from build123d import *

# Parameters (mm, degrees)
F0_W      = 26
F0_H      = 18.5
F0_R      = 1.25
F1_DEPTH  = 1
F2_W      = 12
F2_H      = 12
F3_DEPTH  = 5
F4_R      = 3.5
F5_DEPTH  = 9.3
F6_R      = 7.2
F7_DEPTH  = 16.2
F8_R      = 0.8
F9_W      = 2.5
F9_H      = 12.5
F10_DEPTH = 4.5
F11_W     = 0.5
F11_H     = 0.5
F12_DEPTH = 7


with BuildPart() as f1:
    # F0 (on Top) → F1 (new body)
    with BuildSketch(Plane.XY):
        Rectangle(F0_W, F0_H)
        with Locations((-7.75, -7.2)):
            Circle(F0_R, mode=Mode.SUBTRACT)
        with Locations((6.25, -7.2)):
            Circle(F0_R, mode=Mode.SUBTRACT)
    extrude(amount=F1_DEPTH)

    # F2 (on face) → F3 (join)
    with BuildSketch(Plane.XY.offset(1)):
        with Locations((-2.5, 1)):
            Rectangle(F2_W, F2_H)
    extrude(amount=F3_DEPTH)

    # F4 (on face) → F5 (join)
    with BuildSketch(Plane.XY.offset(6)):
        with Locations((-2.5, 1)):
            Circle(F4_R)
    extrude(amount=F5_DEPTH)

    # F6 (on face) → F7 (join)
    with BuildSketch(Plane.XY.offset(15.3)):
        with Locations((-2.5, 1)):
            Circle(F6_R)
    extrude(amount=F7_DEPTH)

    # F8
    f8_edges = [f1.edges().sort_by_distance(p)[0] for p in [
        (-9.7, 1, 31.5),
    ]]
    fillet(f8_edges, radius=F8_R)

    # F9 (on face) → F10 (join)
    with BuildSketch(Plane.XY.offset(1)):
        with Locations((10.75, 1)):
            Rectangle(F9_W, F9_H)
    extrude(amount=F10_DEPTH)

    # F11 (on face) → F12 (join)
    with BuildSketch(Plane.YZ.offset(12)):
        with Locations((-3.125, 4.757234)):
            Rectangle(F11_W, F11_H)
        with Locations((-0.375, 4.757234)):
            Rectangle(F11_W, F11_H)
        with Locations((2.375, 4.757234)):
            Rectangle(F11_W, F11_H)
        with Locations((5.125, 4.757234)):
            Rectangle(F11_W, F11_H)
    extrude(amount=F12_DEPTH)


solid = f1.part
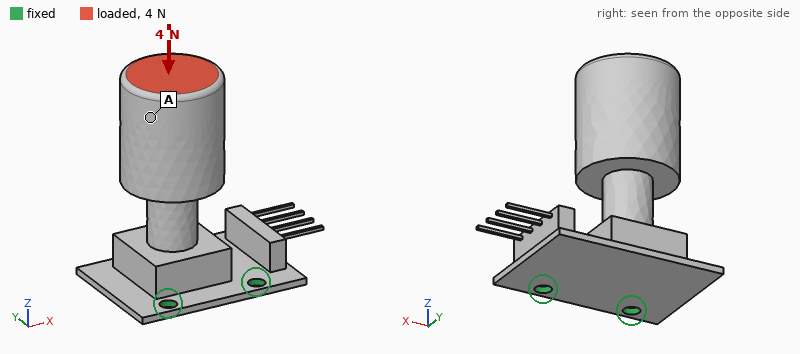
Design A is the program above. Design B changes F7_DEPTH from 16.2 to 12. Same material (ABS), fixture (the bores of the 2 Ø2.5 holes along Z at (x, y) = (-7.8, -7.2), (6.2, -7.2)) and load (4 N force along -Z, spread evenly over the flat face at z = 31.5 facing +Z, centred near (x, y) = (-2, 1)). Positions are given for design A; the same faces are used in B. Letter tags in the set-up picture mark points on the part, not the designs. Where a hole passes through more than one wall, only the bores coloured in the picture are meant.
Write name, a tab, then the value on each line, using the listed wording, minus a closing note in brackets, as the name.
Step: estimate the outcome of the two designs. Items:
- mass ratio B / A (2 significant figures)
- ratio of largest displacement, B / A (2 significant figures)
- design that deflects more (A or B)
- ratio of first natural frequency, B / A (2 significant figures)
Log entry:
mass ratio B / A	0.84
ratio of largest displacement, B / A	0.88
design that deflects more	A
ratio of first natural frequency, B / A	1.3
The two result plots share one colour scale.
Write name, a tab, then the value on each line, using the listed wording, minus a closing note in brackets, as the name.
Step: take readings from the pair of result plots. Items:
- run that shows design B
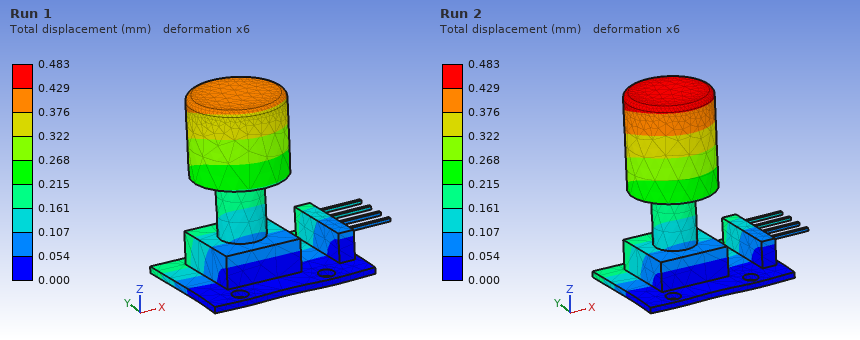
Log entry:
run that shows design B	Run 1
